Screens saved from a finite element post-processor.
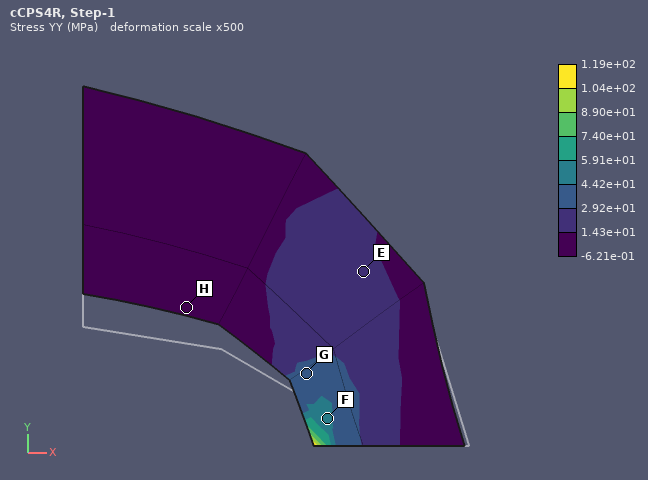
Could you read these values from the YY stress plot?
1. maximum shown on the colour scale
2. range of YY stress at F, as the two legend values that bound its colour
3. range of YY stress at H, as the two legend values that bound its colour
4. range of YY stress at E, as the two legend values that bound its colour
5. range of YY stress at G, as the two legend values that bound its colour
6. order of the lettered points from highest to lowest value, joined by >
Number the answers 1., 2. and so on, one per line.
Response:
1. 1.19e+02 MPa
2. 4.42e+01 to 5.91e+01 MPa
3. -6.21e-01 to 1.43e+01 MPa
4. 1.43e+01 to 2.92e+01 MPa
5. 2.92e+01 to 4.42e+01 MPa
6. F > G > E > H
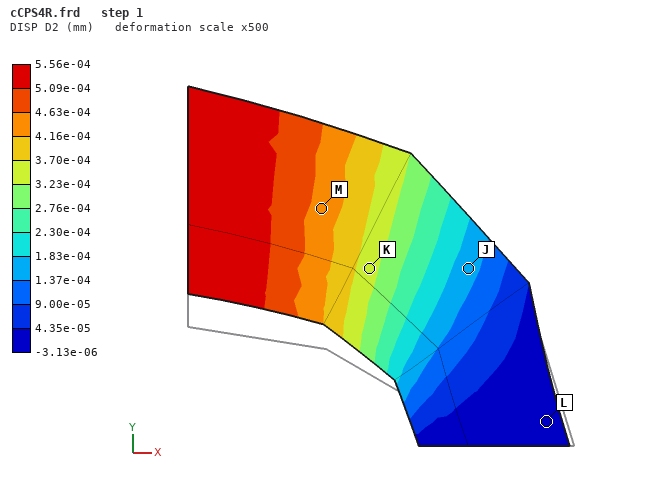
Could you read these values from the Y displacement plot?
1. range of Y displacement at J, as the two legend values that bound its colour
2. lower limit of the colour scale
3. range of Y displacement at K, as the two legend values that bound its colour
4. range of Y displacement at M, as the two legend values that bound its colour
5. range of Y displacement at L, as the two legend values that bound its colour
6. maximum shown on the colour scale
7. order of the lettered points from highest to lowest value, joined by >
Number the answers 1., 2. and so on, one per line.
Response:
1. 1.37e-04 to 1.83e-04 mm
2. -3.13e-06 mm
3. 3.23e-04 to 3.70e-04 mm
4. 4.16e-04 to 4.63e-04 mm
5. -3.13e-06 to 4.35e-05 mm
6. 5.56e-04 mm
7. M > K > J > L
